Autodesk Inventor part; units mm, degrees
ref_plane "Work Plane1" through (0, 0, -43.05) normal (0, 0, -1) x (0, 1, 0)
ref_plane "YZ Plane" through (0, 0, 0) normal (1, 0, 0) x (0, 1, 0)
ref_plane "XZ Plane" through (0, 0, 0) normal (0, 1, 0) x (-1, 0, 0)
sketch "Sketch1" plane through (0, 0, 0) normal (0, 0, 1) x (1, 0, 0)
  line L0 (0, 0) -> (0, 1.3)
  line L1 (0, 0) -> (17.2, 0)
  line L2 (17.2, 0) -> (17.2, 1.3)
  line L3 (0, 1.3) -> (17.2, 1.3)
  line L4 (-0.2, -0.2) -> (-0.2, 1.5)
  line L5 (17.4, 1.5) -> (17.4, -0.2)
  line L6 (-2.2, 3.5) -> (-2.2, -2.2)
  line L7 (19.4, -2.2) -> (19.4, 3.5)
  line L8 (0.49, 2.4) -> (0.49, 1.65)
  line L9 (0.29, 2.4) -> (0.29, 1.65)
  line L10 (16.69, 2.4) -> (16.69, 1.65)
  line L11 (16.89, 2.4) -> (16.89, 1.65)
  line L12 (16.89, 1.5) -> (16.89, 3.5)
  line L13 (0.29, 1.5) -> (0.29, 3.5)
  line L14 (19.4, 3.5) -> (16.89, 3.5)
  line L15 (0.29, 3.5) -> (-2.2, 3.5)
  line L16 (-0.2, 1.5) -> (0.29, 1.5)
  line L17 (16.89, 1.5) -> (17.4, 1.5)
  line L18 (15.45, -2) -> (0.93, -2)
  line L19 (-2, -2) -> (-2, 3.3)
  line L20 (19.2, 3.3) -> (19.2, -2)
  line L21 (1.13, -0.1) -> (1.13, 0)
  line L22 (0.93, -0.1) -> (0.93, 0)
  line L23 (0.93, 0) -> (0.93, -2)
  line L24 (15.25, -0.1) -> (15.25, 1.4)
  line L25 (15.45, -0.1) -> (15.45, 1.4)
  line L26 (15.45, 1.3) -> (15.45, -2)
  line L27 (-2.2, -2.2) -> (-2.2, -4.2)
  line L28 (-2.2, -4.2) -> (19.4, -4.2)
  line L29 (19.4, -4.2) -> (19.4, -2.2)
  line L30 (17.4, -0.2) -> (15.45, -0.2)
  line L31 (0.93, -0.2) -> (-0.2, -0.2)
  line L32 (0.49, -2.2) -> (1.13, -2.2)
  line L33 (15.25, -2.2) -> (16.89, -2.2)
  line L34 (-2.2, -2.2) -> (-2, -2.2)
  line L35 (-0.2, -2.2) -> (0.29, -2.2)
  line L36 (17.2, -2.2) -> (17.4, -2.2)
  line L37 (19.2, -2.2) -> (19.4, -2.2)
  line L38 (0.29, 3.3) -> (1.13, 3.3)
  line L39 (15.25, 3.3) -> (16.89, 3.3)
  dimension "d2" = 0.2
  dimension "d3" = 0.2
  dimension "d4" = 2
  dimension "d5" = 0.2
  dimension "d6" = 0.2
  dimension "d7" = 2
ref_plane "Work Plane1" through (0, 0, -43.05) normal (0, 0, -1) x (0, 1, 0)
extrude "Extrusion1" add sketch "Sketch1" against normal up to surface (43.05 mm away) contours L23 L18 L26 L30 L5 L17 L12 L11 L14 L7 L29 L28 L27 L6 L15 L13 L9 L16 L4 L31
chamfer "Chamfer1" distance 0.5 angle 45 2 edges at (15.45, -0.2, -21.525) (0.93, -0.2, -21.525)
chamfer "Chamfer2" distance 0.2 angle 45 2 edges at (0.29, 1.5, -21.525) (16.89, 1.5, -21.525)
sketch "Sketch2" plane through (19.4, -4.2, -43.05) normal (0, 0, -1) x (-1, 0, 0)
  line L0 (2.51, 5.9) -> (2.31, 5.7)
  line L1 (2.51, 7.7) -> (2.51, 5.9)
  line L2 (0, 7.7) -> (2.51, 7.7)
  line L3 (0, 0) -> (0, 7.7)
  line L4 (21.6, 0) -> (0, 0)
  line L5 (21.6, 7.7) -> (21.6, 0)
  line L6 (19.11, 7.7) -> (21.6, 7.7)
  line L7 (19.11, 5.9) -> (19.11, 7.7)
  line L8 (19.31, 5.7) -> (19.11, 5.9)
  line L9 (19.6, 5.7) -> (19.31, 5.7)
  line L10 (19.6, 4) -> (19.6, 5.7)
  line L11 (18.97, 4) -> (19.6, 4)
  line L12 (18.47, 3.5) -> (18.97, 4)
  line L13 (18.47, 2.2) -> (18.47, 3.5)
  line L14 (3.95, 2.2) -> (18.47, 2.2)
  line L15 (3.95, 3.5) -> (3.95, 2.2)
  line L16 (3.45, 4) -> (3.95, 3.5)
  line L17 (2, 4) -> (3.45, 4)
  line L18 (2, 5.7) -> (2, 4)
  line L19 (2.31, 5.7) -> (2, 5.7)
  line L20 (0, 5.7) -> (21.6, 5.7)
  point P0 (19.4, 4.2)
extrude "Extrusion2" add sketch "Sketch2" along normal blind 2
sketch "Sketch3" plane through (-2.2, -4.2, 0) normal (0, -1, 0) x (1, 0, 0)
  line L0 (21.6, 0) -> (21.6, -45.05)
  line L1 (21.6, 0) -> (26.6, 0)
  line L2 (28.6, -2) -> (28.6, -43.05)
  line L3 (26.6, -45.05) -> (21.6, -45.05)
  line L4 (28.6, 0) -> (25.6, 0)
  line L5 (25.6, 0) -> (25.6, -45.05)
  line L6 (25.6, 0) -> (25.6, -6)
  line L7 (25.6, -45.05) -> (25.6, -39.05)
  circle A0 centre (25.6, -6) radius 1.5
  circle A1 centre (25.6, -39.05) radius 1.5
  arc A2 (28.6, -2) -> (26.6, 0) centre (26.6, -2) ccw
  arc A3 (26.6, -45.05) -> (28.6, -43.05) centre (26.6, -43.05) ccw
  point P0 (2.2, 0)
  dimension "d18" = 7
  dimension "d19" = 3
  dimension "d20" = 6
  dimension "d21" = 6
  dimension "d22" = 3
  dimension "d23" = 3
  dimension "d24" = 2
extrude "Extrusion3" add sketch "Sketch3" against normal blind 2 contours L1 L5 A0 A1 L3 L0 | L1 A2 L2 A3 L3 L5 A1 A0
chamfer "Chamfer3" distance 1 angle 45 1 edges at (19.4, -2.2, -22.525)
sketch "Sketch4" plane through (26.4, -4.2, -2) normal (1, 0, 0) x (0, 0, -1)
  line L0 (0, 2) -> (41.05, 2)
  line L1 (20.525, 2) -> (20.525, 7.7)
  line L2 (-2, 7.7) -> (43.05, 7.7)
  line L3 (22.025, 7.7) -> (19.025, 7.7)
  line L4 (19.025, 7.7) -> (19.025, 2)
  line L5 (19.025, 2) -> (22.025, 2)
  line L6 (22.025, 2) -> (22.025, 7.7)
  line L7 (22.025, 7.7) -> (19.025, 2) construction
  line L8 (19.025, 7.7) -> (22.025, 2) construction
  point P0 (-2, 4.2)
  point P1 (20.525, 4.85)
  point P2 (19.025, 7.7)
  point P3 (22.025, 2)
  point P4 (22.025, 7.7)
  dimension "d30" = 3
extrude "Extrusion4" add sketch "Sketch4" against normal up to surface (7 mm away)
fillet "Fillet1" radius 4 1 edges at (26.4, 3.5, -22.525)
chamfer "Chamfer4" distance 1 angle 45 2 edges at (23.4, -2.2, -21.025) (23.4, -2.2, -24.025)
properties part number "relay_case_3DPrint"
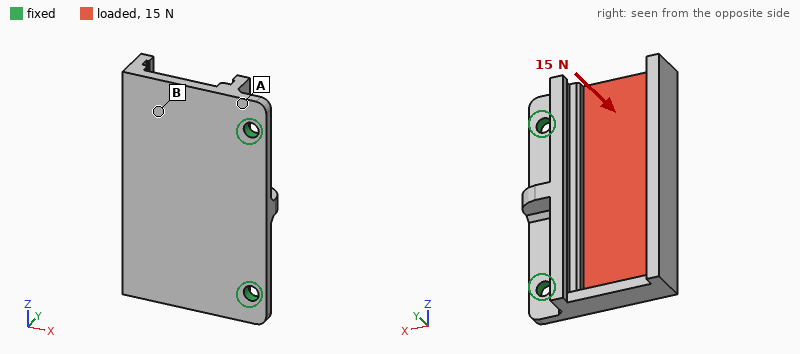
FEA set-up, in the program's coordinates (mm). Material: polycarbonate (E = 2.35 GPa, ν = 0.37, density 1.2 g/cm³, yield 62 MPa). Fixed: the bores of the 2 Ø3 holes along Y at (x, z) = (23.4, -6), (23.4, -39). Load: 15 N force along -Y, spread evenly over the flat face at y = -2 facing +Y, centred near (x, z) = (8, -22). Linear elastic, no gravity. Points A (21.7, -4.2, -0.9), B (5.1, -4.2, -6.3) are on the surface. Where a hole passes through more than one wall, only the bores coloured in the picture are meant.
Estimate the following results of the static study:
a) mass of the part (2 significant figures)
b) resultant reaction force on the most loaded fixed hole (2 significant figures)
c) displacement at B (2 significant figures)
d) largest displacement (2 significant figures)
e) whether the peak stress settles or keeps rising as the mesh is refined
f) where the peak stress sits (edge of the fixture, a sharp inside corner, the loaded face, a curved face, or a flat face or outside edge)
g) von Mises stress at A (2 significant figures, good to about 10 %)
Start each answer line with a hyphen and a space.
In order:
- 5.2 g
- 8.5 N
- 0.31 mm
- 0.50 mm
- keeps rising
- edge of the fixture
- 6.0 MPa
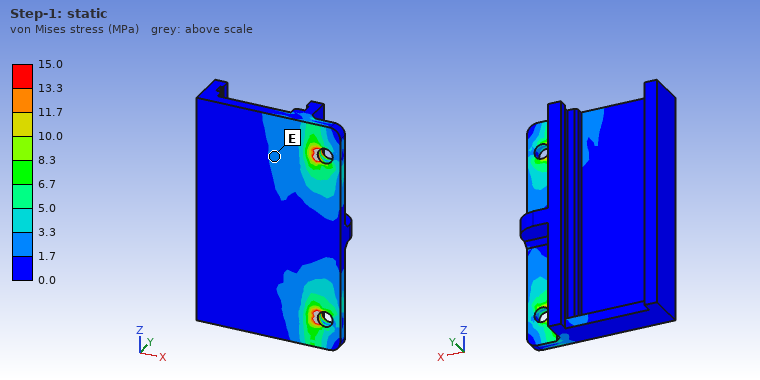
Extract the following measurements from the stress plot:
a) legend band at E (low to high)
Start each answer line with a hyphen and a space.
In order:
- 1.7 to 3.3 MPa
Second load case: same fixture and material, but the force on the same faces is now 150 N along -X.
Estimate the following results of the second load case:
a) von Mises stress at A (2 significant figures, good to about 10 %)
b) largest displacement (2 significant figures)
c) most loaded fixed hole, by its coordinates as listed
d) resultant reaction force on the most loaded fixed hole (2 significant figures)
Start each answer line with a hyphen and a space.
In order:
- 4.5 MPa
- 0.51 mm
- (23.4, -6)
- 81 N
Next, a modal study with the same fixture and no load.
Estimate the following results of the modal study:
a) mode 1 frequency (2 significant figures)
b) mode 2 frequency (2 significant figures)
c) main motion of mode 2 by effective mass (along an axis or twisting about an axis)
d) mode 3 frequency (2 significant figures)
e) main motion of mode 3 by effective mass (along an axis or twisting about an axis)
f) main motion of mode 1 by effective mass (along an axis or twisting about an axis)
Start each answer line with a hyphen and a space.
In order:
- 510 Hz
- 1100 Hz
- twisting about X
- 3100 Hz
- along Y
- along Y
